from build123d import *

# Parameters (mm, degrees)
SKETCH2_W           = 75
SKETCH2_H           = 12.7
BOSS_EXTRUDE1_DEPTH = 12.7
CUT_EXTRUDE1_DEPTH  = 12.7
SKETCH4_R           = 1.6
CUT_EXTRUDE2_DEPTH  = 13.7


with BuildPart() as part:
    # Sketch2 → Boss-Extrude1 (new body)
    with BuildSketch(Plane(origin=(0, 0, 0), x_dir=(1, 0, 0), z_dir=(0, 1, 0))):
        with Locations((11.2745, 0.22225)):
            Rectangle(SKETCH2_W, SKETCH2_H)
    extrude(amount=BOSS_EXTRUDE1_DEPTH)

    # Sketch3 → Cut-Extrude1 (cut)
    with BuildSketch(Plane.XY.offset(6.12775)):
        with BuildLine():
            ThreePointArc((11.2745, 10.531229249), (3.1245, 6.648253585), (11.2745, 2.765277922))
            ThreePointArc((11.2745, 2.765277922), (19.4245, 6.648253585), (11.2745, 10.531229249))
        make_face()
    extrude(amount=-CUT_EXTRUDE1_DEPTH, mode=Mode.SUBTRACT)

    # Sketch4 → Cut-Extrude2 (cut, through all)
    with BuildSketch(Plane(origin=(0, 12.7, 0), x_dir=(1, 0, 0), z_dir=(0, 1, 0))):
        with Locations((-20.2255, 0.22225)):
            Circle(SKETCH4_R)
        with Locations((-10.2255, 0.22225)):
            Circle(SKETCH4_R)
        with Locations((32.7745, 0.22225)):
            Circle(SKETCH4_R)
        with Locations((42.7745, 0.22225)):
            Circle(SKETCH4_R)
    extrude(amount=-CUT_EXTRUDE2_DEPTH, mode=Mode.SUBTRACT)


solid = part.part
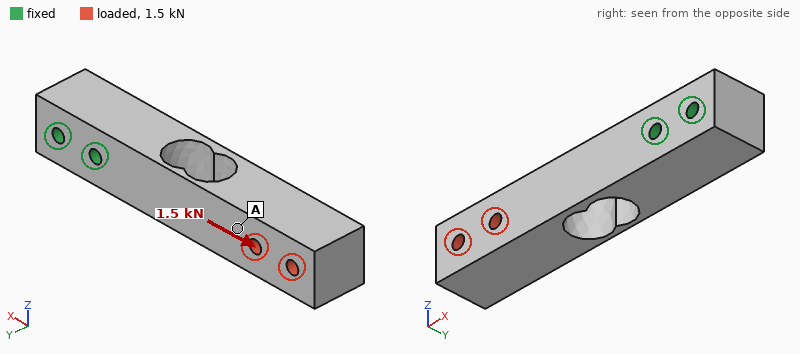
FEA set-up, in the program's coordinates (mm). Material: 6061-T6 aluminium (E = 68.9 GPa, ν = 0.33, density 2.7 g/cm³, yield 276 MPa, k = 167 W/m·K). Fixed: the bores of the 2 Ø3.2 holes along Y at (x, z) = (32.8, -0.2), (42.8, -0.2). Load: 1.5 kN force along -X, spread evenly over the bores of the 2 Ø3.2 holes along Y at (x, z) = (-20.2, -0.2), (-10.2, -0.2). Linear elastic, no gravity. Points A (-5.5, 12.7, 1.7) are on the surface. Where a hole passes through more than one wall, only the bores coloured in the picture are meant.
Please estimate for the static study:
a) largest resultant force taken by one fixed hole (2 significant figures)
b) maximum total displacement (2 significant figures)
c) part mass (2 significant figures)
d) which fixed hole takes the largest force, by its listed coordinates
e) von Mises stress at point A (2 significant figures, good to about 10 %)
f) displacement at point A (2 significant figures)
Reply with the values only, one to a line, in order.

1.3 kN
22 µm
27 g
(32.8, -0.2)
12 MPa
17 µm
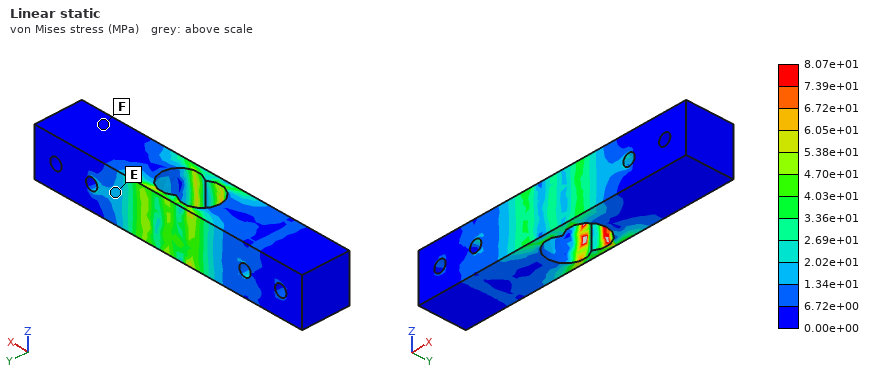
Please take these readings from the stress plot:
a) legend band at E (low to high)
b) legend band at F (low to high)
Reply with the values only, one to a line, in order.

1.34e+01 to 2.02e+01 MPa
0.00e+00 to 6.72e+00 MPa
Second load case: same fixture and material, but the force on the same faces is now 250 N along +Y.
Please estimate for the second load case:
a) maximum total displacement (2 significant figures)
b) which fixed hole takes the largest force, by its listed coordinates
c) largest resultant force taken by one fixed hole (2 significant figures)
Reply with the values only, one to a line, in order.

0.19 mm
(32.8, -0.2)
420 N
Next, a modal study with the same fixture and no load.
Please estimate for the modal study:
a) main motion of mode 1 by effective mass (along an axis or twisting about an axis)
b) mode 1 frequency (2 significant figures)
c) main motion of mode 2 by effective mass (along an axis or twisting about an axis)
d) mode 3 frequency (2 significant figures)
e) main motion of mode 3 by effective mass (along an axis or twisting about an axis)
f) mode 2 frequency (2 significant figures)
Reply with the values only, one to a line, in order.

along Y
1800 Hz
along Z
7400 Hz
twisting about X
1900 Hz
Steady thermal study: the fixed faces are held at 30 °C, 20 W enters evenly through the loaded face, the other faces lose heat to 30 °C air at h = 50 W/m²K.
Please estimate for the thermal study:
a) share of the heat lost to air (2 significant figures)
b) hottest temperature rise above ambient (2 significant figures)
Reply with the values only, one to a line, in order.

28 %
54 K
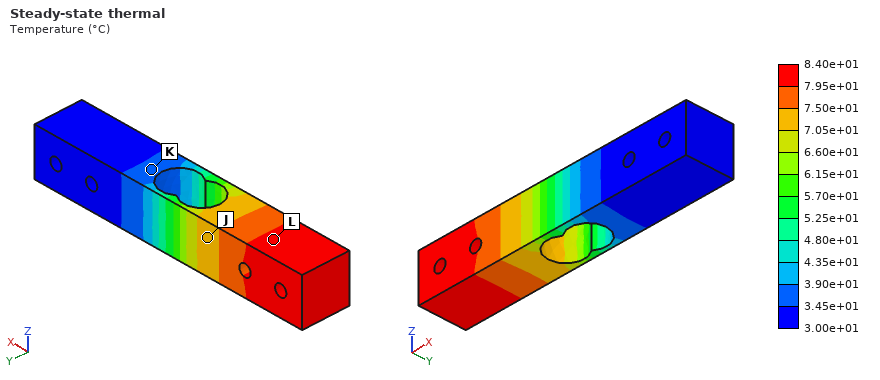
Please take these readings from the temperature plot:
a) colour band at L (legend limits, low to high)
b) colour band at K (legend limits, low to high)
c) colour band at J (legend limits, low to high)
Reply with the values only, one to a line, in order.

7.95e+01 to 8.40e+01 °C
3.45e+01 to 3.90e+01 °C
7.05e+01 to 7.50e+01 °C
